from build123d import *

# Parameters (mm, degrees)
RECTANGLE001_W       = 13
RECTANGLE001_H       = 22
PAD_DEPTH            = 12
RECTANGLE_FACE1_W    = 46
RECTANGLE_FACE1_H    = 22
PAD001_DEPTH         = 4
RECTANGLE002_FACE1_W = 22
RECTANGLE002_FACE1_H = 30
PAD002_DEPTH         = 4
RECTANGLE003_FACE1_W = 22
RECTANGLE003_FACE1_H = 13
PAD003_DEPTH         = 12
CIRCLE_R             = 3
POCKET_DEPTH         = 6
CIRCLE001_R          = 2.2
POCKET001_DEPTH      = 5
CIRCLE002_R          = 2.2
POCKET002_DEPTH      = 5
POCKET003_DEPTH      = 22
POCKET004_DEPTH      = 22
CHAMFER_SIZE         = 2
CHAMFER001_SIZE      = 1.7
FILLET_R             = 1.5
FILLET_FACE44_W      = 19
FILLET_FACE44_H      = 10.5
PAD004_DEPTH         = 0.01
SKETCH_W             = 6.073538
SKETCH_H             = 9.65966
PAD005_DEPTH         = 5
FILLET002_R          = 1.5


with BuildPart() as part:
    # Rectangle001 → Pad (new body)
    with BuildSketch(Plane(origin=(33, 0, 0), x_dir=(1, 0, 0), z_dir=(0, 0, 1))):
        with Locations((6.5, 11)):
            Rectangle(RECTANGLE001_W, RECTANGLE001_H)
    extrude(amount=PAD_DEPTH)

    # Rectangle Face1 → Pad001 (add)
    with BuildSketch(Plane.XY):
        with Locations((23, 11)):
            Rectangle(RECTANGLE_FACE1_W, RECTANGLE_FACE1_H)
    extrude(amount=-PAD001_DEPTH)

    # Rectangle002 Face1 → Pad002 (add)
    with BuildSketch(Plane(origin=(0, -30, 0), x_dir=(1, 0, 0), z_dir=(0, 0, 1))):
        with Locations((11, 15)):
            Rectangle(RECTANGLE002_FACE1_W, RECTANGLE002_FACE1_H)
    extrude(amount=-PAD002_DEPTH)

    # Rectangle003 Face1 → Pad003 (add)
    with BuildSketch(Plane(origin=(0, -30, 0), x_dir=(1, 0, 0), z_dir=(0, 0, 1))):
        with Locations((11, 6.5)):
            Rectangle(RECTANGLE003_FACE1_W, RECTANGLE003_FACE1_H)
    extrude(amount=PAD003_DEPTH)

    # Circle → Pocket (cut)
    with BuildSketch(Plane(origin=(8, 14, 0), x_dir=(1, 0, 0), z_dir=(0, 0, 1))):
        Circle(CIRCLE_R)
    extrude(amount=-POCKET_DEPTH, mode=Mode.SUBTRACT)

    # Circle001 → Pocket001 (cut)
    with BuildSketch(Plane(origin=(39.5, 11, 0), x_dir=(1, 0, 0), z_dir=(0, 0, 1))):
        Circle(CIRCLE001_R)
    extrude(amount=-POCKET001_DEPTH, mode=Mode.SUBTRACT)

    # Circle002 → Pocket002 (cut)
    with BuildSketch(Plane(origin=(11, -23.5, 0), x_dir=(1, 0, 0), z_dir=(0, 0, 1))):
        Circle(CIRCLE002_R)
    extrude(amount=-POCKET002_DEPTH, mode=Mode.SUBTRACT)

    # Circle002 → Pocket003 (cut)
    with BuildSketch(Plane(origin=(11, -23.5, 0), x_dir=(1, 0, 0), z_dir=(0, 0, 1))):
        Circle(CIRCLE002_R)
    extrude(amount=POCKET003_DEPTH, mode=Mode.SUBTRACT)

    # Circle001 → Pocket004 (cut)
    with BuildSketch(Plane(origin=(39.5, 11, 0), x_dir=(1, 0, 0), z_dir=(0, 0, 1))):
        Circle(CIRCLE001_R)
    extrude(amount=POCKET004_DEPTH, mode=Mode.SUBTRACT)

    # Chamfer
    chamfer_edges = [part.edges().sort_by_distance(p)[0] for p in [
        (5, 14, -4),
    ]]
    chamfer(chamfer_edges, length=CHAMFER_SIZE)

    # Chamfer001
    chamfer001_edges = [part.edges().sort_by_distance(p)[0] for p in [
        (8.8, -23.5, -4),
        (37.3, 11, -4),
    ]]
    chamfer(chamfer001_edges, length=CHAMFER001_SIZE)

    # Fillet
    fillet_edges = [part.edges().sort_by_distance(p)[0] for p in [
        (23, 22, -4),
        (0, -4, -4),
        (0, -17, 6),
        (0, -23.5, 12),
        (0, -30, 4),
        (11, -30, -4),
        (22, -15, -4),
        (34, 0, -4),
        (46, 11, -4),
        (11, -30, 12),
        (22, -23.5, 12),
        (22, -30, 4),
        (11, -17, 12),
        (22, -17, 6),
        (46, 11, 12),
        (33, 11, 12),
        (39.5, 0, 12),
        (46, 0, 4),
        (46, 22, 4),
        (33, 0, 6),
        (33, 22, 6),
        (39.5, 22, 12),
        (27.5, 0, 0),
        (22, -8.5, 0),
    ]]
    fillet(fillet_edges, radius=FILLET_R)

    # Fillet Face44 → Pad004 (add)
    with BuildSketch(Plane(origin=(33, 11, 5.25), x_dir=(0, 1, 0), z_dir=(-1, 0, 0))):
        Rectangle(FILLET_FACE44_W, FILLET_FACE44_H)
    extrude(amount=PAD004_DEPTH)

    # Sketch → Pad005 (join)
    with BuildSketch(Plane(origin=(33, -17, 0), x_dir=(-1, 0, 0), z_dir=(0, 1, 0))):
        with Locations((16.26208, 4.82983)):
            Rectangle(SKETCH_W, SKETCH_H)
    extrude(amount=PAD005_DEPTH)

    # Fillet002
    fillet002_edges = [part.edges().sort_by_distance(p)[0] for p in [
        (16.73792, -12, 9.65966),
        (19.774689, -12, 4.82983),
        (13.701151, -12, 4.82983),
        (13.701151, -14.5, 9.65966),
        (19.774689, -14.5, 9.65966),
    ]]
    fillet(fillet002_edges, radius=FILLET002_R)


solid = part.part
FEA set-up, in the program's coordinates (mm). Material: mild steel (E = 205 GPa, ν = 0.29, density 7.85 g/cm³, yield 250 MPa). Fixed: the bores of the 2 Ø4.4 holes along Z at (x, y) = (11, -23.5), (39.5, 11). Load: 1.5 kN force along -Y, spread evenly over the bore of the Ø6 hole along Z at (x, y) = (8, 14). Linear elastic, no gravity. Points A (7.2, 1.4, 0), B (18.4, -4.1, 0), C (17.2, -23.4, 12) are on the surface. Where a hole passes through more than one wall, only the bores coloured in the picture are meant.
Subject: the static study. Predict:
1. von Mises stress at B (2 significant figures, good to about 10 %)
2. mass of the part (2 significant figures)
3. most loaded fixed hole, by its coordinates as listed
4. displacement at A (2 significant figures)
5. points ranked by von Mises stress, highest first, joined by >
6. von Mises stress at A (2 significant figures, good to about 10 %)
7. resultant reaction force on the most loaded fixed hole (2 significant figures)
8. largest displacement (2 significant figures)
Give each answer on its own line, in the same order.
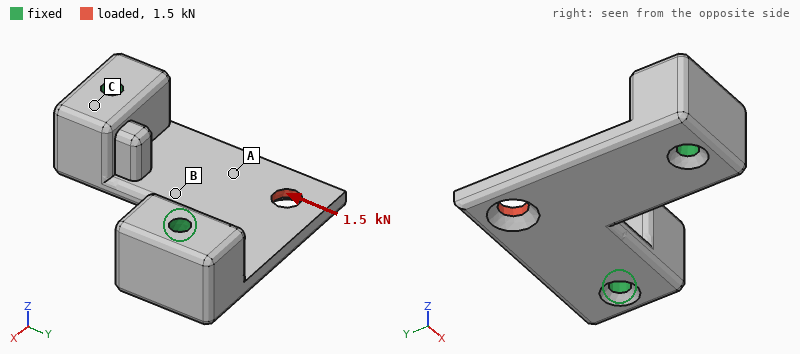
18 MPa
100 g
(11, -23.5)
2.9 µm
A > B > C
32 MPa
1.4 kN
15 µm
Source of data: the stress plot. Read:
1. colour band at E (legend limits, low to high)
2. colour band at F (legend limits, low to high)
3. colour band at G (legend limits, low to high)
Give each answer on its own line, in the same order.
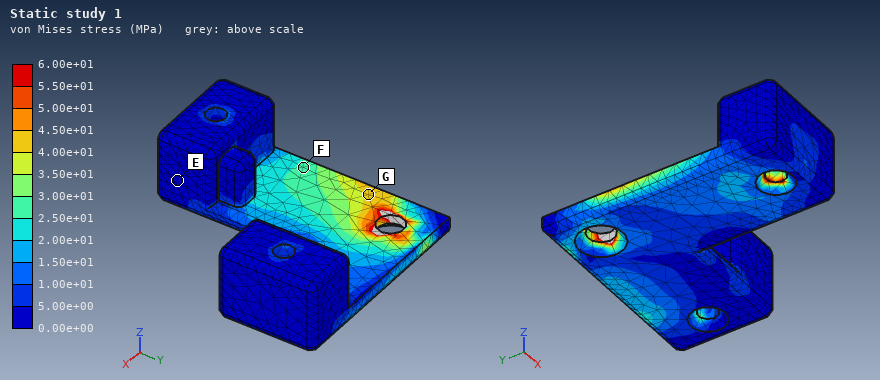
0.00e+00 to 5.00e+00 MPa
2.50e+01 to 3.00e+01 MPa
4.00e+01 to 4.50e+01 MPa
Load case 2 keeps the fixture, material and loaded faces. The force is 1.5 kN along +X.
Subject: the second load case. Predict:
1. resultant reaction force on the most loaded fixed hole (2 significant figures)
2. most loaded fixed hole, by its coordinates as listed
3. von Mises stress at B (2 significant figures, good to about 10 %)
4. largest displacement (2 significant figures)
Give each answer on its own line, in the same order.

1.4 kN
(39.5, 11)
9.4 MPa
16 µm
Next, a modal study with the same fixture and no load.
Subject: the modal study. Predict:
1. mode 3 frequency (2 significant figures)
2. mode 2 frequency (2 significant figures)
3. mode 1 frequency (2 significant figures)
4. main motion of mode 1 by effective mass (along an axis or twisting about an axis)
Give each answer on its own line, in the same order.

17 kHz
14 kHz
4700 Hz
along Z
